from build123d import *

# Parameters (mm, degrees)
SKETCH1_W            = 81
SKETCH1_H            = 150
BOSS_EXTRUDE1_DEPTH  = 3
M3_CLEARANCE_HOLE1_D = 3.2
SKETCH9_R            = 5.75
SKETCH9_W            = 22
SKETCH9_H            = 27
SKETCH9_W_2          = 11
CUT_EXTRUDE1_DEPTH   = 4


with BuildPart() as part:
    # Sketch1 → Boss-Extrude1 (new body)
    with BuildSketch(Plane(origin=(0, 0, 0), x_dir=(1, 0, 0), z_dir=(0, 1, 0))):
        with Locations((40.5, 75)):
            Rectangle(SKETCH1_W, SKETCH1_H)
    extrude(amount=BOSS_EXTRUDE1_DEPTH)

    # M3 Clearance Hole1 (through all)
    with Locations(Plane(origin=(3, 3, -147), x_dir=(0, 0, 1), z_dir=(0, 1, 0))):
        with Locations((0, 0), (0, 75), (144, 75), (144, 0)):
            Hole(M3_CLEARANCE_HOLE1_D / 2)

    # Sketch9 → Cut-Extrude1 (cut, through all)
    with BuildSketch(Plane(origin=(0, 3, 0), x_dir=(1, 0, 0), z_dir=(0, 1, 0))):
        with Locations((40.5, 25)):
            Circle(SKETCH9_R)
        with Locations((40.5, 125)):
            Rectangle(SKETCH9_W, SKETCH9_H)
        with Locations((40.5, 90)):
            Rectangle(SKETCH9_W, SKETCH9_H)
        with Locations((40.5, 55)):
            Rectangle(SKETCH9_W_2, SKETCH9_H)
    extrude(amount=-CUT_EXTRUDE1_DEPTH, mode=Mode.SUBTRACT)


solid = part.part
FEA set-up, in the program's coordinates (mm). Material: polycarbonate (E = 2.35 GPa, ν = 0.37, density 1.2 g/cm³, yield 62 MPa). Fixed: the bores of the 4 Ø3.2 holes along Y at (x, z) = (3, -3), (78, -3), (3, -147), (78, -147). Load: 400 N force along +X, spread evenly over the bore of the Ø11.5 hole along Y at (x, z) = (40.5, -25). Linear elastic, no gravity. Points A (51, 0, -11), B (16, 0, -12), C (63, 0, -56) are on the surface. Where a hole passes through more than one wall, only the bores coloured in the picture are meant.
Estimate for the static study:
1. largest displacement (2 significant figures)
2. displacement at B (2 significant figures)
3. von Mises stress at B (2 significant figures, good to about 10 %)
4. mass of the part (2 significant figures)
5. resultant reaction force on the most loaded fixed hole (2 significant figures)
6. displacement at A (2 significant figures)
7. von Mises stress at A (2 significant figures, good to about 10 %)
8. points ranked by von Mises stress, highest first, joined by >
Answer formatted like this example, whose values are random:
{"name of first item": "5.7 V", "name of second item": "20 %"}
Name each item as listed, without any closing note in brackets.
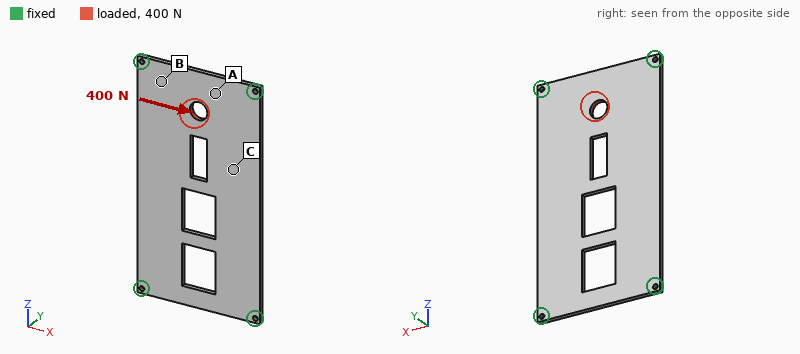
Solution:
{"largest displacement": "96 µm", "displacement at B": "46 µm", "von Mises stress at B": "3.5 MPa", "mass of the part": "38 g", "resultant reaction force on the most loaded fixed hole": "200 N", "displacement at A": "52 µm", "von Mises stress at A": "2.6 MPa", "points ranked by von Mises stress, highest first, joined by >": "B > A > C"}
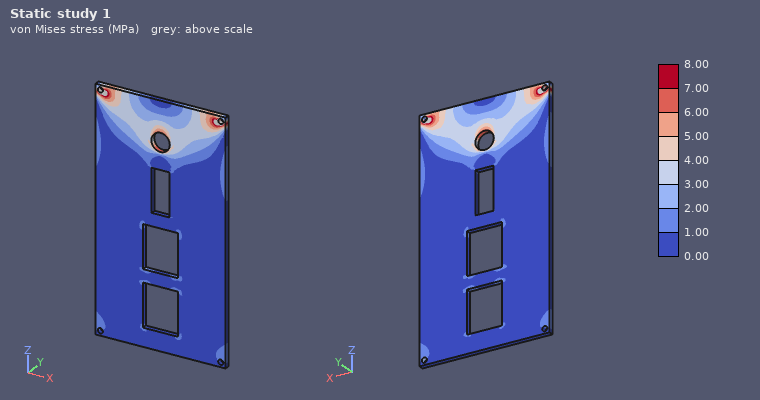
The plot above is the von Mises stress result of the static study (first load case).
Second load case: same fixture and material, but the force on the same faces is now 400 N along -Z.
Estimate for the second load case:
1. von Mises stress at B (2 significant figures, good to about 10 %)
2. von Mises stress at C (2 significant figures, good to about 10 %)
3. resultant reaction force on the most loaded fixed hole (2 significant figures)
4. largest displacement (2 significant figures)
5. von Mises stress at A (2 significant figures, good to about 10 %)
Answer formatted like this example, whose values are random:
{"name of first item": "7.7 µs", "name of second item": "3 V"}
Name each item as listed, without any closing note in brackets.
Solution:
{"von Mises stress at B": "2.4 MPa", "von Mises stress at C": "1.2 MPa", "resultant reaction force on the most loaded fixed hole": "150 N", "largest displacement": "97 µm", "von Mises stress at A": "2.2 MPa"}
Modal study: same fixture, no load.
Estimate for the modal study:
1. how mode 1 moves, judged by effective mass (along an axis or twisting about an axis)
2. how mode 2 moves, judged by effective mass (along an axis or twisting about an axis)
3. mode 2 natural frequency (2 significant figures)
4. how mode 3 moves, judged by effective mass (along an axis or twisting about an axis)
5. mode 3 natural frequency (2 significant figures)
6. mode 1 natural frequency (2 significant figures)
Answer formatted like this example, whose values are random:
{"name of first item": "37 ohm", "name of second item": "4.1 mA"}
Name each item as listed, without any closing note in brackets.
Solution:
{"how mode 1 moves, judged by effective mass": "along Y", "how mode 2 moves, judged by effective mass": "twisting about Z", "mode 2 natural frequency": "290 Hz", "how mode 3 moves, judged by effective mass": "twisting about X", "mode 3 natural frequency": "450 Hz", "mode 1 natural frequency": "160 Hz"}
